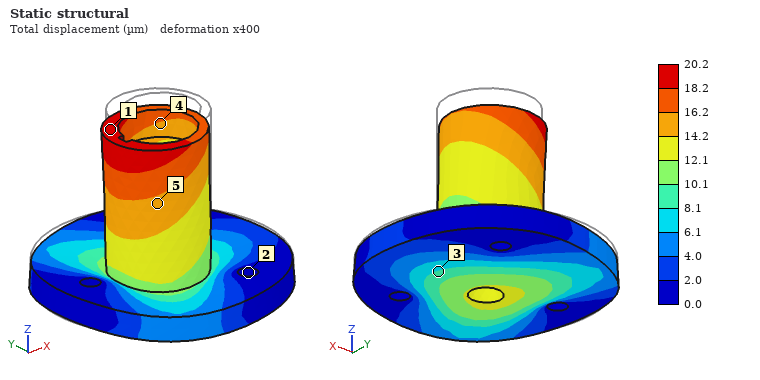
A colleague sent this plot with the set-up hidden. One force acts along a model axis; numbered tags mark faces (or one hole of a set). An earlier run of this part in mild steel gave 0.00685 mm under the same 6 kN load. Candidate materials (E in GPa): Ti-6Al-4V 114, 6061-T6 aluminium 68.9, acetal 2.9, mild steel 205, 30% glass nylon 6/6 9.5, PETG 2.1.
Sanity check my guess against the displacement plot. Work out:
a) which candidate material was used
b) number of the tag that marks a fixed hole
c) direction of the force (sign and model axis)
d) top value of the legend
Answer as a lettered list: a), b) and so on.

a) 6061-T6 aluminium
b) 2
c) -Z
d) 20.2 µm
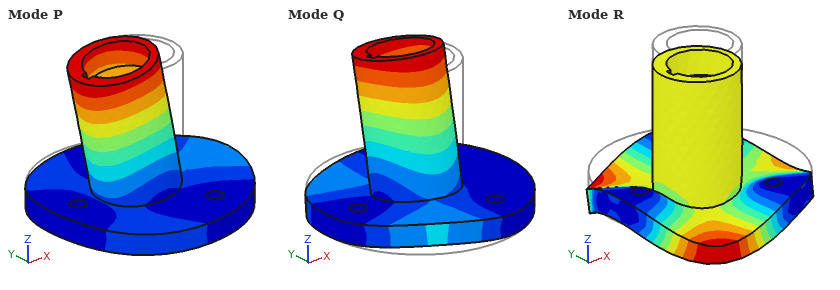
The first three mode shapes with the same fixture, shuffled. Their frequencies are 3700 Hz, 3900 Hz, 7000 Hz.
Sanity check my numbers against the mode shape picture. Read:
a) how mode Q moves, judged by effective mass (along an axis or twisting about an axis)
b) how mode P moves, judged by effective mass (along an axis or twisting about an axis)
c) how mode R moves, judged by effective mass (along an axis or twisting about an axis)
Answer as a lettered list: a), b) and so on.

a) along Y
b) along X
c) along Z
